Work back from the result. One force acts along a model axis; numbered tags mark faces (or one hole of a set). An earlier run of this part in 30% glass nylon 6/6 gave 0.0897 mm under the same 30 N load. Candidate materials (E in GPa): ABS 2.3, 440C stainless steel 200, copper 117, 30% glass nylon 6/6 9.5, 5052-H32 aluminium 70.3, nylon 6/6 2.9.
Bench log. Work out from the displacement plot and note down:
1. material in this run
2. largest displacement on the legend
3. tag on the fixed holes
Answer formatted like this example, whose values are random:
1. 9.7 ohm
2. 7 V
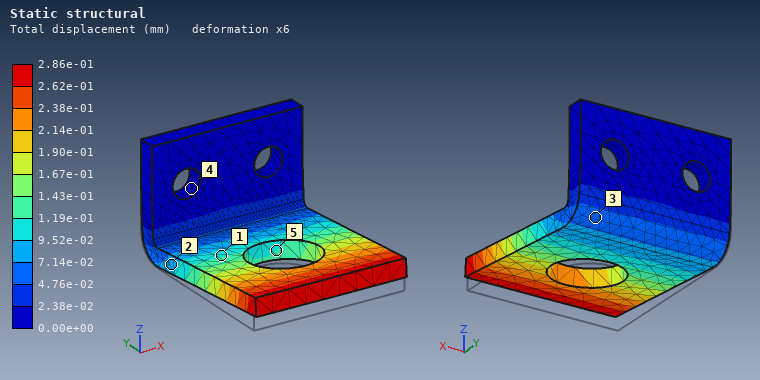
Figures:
1. nylon 6/6
2. 2.86e-01 mm
3. 4
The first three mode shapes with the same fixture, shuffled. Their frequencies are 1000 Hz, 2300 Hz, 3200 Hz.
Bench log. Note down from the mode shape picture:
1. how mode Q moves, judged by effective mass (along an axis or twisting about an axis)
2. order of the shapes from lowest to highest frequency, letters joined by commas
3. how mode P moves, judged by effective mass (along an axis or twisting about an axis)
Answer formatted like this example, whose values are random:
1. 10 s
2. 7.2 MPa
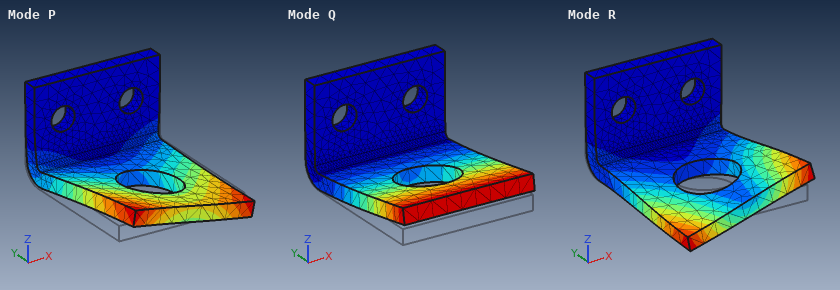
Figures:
1. along Z
2. Q, P, R
3. along X
